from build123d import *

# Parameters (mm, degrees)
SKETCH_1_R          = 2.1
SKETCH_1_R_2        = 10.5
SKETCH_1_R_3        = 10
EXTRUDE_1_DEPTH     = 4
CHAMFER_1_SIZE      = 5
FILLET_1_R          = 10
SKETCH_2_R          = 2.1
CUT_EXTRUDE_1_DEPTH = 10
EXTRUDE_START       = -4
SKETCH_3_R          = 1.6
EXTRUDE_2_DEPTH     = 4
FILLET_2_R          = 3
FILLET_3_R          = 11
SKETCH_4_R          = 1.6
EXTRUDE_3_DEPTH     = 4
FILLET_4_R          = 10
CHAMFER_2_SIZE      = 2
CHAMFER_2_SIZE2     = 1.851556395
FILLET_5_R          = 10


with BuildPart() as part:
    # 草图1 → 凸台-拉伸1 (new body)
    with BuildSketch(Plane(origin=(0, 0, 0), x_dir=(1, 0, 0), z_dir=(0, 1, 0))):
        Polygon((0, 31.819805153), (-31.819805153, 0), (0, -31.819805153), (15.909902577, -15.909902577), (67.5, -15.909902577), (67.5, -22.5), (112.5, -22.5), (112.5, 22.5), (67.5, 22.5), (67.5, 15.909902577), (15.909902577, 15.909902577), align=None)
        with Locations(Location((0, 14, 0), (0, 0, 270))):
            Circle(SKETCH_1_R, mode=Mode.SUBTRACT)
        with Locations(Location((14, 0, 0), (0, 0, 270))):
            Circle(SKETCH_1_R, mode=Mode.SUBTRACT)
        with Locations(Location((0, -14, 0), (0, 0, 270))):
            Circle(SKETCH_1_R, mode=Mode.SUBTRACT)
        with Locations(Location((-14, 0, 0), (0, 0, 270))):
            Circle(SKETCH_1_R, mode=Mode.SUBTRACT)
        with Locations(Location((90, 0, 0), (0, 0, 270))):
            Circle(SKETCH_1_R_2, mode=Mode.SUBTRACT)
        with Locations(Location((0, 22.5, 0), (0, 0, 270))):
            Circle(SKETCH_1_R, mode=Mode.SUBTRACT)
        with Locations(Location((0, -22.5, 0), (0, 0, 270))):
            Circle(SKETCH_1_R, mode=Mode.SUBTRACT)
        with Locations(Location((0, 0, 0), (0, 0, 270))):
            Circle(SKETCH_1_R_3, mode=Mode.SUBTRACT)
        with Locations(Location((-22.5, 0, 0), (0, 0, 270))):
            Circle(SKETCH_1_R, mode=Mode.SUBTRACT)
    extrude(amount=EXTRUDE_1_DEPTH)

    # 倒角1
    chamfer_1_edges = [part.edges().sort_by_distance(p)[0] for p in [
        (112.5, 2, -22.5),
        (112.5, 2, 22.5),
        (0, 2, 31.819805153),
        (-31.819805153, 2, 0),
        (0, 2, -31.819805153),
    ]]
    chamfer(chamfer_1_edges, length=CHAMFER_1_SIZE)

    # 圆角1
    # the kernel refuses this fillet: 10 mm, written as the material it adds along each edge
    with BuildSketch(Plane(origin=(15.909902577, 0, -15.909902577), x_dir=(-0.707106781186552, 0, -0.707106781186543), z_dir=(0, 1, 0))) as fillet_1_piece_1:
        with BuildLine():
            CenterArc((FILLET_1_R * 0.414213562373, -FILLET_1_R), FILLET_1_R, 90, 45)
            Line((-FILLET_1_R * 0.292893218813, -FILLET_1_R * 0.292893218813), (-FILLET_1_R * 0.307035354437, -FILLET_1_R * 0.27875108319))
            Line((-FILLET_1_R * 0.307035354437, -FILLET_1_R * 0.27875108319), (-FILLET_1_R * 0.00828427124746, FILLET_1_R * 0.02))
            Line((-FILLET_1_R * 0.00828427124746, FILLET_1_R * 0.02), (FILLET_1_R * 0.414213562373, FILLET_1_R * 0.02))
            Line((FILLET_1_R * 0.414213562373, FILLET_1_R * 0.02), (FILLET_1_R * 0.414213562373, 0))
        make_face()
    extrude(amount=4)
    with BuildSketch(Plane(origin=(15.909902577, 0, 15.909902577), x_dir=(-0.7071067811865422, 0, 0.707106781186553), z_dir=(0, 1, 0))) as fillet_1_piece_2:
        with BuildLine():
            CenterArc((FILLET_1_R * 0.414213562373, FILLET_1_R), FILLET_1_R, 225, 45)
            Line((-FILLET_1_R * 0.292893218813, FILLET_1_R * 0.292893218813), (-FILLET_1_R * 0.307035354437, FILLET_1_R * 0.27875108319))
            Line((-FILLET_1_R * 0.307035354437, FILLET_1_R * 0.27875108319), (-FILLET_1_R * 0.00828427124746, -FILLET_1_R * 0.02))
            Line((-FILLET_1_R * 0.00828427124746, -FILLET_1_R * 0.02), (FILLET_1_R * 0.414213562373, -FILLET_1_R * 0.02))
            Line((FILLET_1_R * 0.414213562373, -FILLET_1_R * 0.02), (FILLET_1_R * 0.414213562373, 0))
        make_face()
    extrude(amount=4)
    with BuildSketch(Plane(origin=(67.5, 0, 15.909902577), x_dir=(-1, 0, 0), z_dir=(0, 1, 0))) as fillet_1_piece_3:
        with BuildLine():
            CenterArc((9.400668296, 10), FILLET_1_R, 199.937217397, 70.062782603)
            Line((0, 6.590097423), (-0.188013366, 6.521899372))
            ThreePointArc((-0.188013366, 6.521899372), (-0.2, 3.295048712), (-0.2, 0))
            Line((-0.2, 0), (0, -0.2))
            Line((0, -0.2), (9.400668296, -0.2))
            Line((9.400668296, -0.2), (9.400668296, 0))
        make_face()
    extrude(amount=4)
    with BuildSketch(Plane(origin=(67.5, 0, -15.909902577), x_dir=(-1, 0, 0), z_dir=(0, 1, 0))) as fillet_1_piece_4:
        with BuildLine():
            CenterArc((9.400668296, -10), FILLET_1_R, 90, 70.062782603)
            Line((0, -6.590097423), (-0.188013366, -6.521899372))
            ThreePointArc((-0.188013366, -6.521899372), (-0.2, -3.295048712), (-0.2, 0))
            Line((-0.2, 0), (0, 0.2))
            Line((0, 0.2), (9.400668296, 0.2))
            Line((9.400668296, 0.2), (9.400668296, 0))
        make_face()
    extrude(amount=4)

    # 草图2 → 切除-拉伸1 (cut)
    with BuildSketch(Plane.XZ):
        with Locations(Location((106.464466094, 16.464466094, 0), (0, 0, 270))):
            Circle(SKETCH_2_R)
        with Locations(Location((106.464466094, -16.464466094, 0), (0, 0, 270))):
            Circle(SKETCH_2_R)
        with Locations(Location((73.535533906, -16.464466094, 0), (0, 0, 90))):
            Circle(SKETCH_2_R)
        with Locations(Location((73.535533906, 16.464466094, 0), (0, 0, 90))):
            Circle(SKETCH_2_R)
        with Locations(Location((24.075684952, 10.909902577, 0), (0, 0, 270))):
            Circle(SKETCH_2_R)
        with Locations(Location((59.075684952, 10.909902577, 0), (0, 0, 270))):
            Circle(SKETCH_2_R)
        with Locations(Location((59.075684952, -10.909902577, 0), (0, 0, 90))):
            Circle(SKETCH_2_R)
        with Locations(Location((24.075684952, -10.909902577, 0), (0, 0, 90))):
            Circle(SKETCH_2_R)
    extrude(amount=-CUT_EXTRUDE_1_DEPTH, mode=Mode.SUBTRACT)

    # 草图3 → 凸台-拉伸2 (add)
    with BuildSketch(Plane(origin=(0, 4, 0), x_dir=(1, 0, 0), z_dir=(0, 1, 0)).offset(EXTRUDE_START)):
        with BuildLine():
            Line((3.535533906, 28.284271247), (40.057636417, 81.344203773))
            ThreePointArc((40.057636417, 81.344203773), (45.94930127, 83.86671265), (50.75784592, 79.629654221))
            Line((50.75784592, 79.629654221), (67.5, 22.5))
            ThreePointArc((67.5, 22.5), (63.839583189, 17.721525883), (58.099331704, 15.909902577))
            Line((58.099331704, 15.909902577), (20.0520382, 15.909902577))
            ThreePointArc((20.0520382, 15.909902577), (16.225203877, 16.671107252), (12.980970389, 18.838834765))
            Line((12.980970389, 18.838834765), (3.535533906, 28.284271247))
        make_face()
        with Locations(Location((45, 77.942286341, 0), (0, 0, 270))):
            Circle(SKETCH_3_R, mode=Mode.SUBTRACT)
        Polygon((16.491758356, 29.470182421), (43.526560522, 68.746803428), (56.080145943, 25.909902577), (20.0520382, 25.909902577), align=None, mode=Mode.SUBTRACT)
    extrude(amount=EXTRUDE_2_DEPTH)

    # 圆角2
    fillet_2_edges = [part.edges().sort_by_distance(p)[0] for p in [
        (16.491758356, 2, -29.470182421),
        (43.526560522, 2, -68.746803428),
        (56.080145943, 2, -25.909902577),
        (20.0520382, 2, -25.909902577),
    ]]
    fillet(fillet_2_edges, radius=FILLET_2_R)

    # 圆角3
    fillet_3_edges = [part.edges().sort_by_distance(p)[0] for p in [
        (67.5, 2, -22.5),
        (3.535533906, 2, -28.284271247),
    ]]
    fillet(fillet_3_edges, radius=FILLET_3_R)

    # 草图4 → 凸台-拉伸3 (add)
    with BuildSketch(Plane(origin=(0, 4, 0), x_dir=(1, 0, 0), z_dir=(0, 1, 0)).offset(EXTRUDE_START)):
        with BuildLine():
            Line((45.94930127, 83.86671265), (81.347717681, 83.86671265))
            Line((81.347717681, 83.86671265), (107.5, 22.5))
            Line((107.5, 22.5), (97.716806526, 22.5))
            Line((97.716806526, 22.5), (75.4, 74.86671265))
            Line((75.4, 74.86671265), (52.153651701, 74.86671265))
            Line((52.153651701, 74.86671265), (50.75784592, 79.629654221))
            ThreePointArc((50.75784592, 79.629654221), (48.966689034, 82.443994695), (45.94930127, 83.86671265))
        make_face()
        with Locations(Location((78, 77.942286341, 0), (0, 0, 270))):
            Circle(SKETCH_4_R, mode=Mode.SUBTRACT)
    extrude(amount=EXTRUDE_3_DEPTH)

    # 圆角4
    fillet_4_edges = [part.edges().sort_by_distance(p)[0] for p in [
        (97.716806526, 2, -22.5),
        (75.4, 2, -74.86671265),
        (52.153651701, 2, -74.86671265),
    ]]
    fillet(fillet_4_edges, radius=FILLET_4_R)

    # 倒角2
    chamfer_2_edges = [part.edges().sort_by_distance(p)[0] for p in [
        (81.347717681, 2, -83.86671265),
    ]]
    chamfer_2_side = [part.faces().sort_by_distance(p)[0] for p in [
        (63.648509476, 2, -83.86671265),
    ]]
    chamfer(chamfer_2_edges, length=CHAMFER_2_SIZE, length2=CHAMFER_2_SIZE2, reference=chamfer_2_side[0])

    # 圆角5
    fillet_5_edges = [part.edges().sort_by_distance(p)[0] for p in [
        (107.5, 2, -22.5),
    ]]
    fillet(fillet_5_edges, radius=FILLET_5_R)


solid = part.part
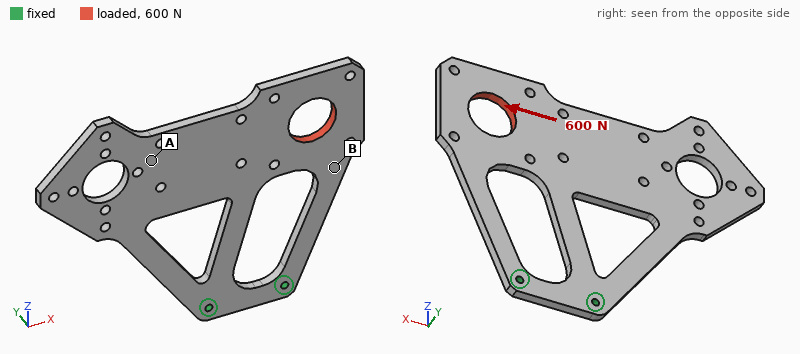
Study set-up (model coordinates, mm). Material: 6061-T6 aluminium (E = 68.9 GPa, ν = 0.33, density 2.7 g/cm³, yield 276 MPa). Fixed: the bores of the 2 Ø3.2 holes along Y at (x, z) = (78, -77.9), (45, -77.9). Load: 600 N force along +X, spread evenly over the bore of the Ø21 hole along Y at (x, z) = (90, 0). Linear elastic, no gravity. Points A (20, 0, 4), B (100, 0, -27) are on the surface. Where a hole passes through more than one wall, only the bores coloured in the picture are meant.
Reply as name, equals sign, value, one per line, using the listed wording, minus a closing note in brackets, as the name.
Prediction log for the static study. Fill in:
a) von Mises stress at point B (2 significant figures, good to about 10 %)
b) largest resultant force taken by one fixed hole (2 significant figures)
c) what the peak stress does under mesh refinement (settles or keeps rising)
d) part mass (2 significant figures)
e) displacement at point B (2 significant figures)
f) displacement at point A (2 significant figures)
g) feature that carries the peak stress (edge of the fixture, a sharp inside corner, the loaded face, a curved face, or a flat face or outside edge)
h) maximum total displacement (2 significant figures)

von Mises stress at point B = 17 MPa
largest resultant force taken by one fixed hole = 1.4 kN
what the peak stress does under mesh refinement = keeps rising
part mass = 78 g
displacement at point B = 0.22 mm
displacement at point A = 0.27 mm
feature that carries the peak stress = edge of the fixture
maximum total displacement = 0.36 mm
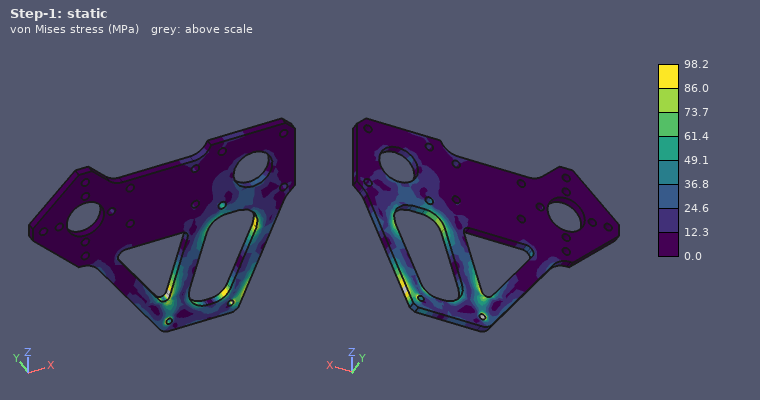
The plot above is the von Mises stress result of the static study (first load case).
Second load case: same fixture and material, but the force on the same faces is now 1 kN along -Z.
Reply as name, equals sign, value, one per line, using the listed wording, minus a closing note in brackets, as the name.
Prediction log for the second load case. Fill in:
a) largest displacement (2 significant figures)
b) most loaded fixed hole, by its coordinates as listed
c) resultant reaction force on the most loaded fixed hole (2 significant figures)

largest displacement = 0.21 mm
most loaded fixed hole, by its coordinates as listed = (78, -77.9)
resultant reaction force on the most loaded fixed hole = 1.3 kN
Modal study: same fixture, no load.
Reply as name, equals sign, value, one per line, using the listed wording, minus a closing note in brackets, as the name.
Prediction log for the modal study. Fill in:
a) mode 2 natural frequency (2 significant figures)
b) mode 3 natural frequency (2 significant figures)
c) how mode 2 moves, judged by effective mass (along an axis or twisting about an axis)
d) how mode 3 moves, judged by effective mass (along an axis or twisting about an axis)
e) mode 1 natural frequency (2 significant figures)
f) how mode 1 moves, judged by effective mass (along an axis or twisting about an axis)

mode 2 natural frequency = 330 Hz
mode 3 natural frequency = 950 Hz
how mode 2 moves, judged by effective mass = twisting about Z
how mode 3 moves, judged by effective mass = along X
mode 1 natural frequency = 170 Hz
how mode 1 moves, judged by effective mass = along Y
